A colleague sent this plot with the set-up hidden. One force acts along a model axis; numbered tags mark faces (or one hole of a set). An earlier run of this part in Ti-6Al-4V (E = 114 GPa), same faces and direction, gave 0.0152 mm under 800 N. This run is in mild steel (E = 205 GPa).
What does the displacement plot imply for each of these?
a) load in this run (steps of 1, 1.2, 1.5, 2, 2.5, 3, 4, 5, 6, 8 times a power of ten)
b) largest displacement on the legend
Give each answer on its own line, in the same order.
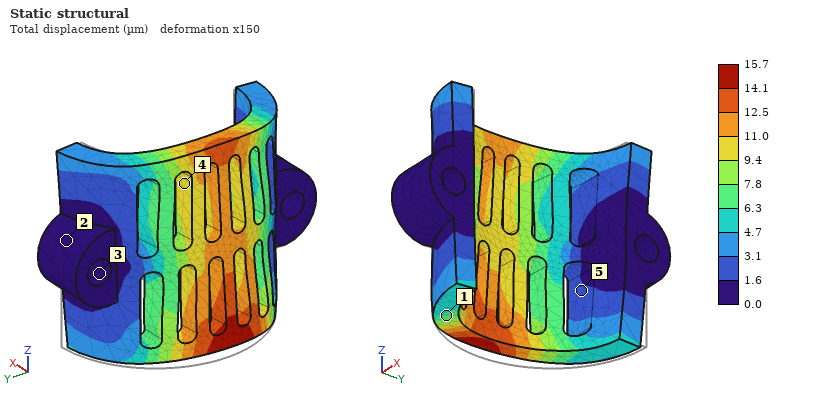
1.5 kN
15.7 µm
